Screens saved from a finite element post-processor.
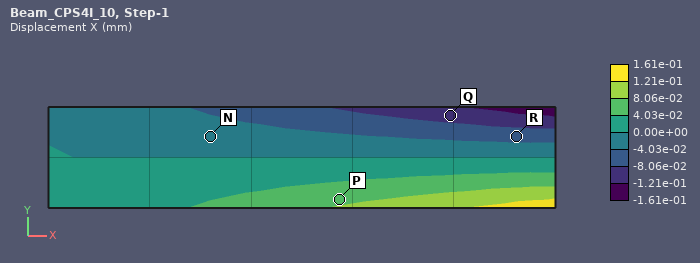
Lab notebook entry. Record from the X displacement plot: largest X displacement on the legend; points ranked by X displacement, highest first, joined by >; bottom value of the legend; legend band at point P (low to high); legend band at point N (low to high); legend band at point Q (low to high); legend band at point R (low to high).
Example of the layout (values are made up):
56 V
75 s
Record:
1.61e-01 mm
P > N > R > Q
-1.61e-01 mm
4.03e-02 to 8.06e-02 mm
-4.03e-02 to 0.00e+00 mm
-1.21e-01 to -8.06e-02 mm
-8.06e-02 to -4.03e-02 mm
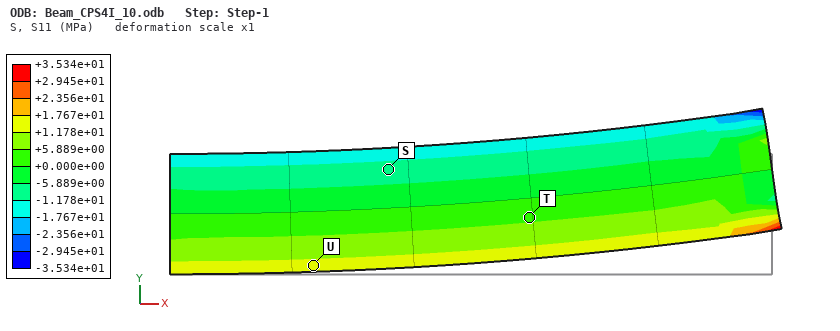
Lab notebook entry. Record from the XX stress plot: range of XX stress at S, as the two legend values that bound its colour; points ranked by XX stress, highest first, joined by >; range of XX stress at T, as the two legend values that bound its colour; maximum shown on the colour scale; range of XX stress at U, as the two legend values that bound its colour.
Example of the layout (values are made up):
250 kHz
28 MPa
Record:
-1.178e+01 to -5.889e+00 MPa
U > T > S
+0.000e+00 to +5.889e+00 MPa
+3.534e+01 MPa
+1.178e+01 to +1.767e+01 MPa
